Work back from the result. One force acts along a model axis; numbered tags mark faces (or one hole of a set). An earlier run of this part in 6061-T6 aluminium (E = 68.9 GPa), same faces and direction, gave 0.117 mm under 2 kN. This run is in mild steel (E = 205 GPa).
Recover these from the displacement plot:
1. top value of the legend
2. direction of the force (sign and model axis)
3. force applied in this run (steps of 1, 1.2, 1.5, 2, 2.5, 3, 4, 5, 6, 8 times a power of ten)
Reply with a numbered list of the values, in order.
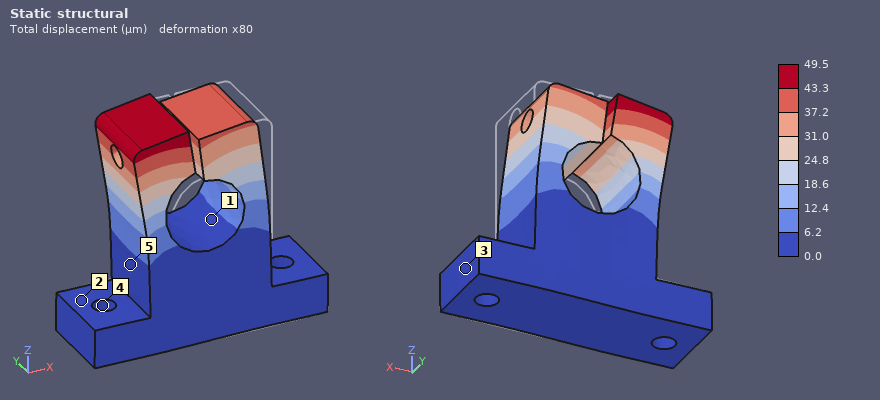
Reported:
1. 49.5 µm
2. -X
3. 2.5 kN
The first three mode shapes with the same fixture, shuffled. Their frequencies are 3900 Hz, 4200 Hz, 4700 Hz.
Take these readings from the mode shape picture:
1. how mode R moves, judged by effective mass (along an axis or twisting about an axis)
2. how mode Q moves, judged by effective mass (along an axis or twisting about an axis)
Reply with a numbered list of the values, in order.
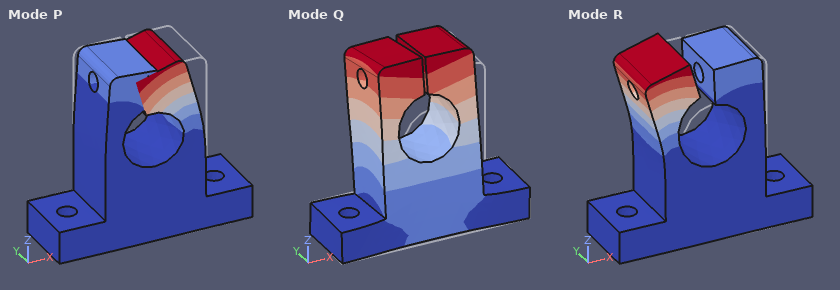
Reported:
1. along X
2. along Y
